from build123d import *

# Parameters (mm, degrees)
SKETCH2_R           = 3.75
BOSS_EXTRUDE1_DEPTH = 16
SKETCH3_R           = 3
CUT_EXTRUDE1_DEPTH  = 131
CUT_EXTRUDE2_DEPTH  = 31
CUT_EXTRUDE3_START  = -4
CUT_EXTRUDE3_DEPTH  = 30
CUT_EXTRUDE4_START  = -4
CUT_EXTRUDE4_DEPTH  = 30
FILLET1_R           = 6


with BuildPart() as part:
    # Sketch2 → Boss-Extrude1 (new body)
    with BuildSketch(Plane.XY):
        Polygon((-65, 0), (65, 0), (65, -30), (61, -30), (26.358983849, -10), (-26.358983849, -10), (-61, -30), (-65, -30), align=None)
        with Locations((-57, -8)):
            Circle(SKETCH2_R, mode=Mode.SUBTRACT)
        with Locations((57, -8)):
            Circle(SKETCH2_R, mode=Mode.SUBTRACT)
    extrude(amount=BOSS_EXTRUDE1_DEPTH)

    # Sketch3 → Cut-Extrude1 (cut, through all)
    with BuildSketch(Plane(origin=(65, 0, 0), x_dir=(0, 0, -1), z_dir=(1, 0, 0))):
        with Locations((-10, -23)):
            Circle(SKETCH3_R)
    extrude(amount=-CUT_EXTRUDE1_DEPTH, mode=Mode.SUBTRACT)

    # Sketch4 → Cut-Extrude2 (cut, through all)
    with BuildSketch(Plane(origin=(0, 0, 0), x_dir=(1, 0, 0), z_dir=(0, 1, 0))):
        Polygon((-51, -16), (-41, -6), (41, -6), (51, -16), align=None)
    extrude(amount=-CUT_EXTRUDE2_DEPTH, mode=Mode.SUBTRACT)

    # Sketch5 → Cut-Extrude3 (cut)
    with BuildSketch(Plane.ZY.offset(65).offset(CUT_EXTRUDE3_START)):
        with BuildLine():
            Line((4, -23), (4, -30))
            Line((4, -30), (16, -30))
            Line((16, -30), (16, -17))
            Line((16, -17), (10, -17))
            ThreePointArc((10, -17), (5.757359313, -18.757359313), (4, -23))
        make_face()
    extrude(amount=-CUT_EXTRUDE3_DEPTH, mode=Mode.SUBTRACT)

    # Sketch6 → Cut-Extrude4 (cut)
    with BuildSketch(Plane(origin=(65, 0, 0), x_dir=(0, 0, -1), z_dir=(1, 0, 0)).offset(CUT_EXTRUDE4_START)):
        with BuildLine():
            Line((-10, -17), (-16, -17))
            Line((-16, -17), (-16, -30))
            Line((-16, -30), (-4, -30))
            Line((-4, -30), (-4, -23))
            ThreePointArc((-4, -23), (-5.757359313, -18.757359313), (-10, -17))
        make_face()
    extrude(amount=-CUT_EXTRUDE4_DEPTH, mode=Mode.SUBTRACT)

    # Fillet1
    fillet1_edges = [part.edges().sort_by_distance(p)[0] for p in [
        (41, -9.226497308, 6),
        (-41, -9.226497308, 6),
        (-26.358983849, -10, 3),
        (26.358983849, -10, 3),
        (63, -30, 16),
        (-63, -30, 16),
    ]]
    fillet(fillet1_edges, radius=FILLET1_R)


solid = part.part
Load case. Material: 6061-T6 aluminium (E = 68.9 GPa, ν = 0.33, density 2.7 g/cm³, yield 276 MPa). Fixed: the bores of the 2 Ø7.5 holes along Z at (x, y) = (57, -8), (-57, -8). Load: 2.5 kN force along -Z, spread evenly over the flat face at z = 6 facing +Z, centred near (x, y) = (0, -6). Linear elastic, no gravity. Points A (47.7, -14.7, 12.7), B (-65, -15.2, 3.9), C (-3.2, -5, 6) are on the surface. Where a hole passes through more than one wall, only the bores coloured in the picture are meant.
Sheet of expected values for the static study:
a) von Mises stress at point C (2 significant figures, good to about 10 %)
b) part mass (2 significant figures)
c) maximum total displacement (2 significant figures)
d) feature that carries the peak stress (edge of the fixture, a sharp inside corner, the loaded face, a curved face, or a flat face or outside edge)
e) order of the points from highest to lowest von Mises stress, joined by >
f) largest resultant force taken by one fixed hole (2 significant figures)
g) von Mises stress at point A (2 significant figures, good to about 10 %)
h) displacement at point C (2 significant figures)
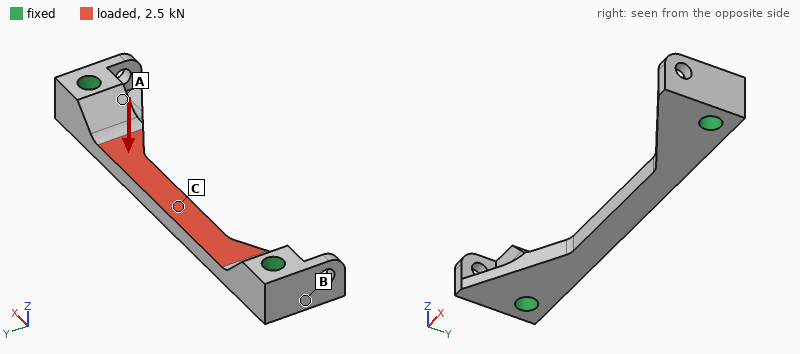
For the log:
130 MPa
50 g
0.35 mm
a curved face
C > A > B
1.4 kN
32 MPa
0.33 mm
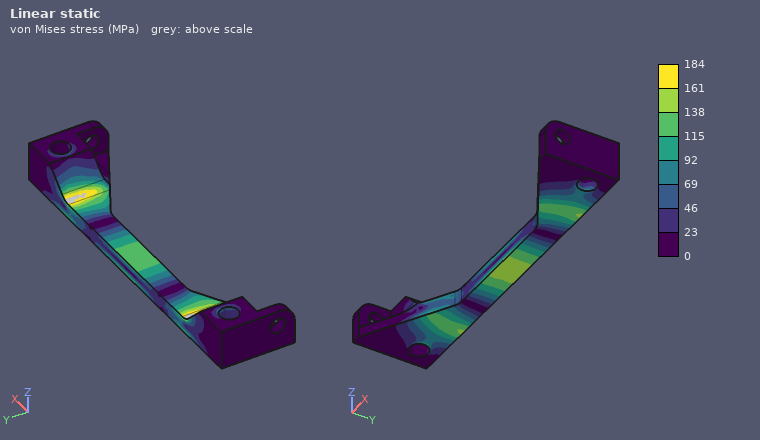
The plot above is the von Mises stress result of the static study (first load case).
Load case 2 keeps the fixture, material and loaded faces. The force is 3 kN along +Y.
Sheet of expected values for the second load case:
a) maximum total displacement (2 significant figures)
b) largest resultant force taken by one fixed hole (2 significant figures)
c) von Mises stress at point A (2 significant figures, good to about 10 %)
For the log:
0.16 mm
1.7 kN
19 MPa
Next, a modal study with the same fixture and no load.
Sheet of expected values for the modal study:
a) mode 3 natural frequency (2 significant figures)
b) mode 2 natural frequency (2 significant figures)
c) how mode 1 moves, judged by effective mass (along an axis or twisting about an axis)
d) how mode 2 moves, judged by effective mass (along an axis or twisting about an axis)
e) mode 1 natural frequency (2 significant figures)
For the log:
10 kHz
7200 Hz
along Z
along Y
4200 Hz
